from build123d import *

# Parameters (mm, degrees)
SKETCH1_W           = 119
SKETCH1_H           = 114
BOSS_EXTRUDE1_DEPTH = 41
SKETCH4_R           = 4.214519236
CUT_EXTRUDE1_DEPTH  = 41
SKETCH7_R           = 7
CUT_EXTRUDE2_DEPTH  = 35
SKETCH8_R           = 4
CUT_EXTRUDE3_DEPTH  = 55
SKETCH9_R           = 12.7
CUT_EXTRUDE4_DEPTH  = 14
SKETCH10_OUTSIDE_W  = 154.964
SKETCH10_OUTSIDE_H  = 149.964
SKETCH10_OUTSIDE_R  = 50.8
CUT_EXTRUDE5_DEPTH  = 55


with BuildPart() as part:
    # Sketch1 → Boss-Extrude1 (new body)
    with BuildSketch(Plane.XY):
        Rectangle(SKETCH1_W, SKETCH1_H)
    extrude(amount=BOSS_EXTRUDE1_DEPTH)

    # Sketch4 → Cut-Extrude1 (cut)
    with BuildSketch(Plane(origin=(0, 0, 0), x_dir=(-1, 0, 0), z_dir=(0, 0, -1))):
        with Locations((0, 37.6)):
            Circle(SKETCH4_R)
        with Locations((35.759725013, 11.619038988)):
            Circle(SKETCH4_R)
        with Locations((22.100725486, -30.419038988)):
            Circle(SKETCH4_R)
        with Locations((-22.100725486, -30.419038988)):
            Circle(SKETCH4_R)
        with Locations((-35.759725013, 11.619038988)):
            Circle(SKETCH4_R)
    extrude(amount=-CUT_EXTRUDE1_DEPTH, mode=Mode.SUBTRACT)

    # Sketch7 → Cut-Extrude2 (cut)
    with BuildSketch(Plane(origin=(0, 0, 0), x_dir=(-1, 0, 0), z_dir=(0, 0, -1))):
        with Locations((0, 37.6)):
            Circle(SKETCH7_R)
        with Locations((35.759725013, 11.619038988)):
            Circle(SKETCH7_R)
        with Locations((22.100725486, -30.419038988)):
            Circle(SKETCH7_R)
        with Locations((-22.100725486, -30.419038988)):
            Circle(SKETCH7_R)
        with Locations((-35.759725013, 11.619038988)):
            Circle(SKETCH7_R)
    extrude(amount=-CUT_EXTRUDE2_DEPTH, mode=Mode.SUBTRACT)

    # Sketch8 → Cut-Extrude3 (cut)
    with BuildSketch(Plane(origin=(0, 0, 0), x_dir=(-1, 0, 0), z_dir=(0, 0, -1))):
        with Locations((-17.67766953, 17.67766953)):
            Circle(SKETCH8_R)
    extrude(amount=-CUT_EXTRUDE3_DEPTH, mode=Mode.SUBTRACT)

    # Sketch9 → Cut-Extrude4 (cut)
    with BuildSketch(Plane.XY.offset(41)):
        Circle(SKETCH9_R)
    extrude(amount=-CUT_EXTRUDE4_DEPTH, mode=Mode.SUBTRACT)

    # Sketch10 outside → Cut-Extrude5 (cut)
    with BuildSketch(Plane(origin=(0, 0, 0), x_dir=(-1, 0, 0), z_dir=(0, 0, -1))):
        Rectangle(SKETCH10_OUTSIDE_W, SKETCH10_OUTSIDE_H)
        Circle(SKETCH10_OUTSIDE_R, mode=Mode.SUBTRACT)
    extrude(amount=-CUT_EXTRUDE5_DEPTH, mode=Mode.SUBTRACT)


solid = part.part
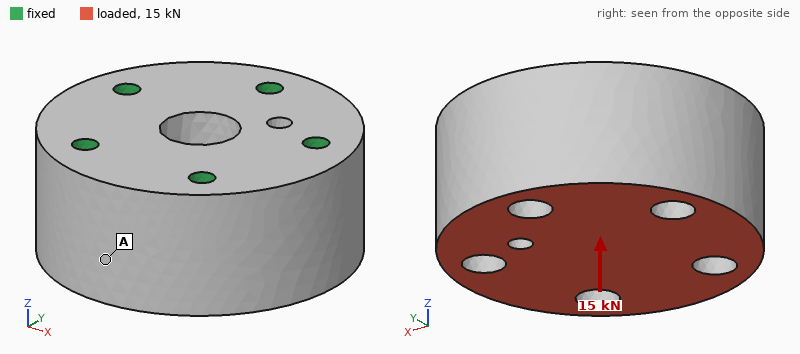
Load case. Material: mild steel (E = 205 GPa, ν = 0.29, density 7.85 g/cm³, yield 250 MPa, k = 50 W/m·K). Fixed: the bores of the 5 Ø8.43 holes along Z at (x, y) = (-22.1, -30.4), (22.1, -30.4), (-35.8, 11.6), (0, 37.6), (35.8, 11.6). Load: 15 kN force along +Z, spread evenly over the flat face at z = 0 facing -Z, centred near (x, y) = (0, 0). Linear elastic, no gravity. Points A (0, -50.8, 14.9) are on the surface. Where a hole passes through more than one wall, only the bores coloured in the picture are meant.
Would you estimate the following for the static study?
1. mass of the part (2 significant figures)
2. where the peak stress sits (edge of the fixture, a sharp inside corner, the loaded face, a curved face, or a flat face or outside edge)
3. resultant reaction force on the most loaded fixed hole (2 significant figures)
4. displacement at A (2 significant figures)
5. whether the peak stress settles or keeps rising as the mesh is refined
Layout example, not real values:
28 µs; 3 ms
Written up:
2.3 kg; edge of the fixture; 3.1 kN; 1.6 µm; keeps rising
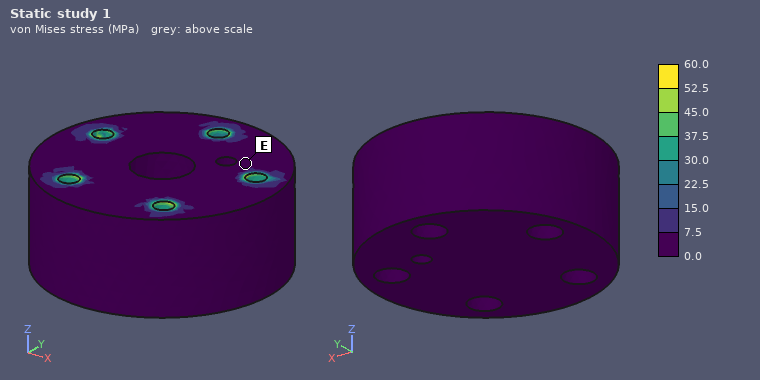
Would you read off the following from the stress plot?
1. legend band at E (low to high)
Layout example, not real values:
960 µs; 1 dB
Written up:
0.0 to 7.5 MPa
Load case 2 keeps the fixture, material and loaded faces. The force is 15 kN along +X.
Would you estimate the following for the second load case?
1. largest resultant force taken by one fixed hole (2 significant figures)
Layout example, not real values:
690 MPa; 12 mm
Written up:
6.4 kN
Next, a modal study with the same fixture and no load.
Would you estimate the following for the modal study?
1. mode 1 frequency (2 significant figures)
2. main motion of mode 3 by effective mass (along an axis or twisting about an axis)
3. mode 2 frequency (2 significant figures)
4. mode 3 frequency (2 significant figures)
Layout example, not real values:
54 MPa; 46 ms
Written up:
7700 Hz; along Z; 7800 Hz; 11 kHz
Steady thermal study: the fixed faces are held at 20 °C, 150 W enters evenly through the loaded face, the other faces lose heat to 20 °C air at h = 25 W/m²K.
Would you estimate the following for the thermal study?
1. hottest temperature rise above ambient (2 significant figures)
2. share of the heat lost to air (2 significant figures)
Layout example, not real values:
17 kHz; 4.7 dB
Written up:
31 K; 9.8 %
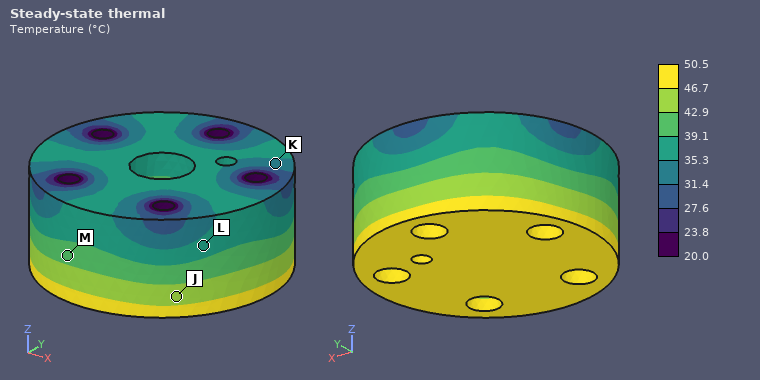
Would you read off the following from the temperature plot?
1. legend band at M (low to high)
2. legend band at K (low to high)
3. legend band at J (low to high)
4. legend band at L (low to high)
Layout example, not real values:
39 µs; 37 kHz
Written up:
39.1 to 42.9 °C; 31.4 to 35.3 °C; 42.9 to 46.7 °C; 35.3 to 39.1 °C
